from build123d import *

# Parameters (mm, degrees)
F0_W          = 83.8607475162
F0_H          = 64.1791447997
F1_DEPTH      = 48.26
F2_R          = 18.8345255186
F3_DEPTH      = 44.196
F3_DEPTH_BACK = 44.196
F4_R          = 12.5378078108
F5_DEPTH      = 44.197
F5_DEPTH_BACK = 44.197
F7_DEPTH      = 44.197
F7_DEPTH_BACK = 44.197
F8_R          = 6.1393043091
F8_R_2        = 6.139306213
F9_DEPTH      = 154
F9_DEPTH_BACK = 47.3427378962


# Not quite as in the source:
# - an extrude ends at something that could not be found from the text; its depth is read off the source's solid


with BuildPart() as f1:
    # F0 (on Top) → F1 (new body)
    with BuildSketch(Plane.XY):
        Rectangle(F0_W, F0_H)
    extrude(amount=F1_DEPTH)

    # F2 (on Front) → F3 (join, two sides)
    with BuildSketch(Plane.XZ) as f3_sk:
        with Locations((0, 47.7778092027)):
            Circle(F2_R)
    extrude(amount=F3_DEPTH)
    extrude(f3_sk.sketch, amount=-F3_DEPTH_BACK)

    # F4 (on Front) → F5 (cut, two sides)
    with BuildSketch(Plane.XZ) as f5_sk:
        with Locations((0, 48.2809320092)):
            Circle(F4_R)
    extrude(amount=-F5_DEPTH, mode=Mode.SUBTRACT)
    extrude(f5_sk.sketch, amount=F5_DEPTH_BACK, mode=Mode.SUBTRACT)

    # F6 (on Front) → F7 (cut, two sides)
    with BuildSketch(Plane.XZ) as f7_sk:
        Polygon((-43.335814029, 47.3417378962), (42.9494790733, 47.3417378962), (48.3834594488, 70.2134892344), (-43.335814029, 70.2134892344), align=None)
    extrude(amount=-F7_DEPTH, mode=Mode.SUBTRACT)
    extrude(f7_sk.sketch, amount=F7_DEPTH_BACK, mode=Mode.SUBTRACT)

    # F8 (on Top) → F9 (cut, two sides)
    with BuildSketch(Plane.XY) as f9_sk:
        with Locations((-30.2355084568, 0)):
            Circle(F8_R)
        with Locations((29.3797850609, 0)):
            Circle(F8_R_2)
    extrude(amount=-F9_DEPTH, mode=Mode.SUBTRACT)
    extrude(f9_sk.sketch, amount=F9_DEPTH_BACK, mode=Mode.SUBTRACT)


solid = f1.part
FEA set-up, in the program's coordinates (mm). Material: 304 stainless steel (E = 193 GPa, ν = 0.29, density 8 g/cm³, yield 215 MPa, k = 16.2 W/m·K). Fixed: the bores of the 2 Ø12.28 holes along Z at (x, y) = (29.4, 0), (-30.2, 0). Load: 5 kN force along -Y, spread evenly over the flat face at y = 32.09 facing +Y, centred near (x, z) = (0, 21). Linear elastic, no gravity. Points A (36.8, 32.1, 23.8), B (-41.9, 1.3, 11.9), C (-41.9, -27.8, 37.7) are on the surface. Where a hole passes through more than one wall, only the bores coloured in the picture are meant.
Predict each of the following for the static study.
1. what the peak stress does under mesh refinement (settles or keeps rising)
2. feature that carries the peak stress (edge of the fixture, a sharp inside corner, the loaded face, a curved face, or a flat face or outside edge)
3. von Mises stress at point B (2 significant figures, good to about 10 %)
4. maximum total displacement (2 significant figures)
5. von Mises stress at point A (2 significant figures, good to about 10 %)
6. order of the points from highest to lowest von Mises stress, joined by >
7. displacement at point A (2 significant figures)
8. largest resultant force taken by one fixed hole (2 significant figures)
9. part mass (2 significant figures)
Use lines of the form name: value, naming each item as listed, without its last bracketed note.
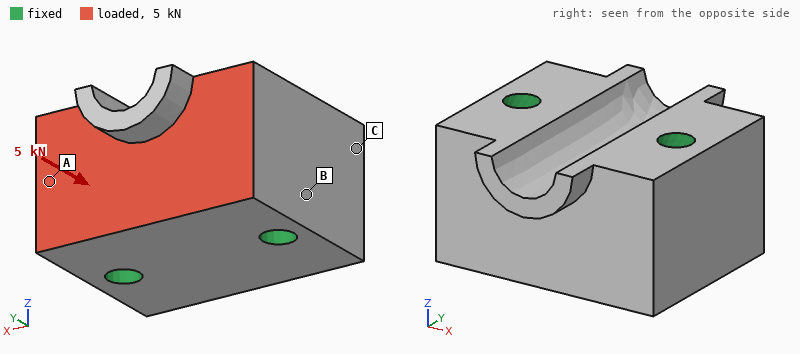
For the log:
what the peak stress does under mesh refinement: keeps rising
feature that carries the peak stress: edge of the fixture
von Mises stress at point B: 0.87 MPa
maximum total displacement: 0.39 µm
von Mises stress at point A: 1.5 MPa
order of the points from highest to lowest von Mises stress, joined by >: A > B > C
displacement at point A: 0.23 µm
largest resultant force taken by one fixed hole: 2.5 kN
part mass: 1.9 kg
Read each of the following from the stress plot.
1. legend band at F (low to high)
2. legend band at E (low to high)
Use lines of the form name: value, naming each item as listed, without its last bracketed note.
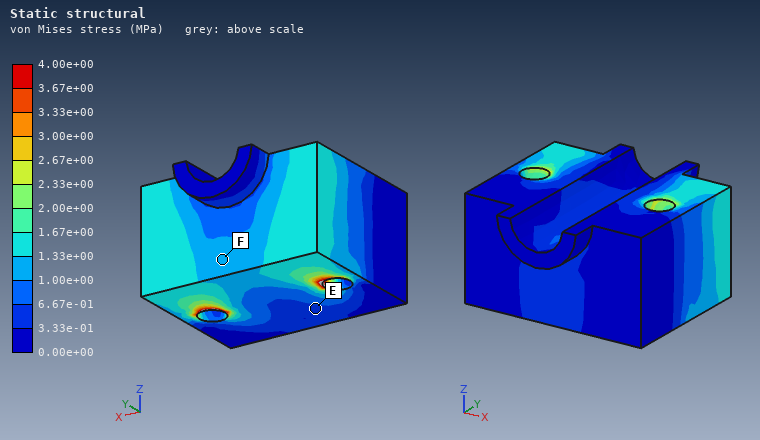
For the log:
legend band at F: 1.00e+00 to 1.33e+00 MPa
legend band at E: 3.33e-01 to 6.67e-01 MPa
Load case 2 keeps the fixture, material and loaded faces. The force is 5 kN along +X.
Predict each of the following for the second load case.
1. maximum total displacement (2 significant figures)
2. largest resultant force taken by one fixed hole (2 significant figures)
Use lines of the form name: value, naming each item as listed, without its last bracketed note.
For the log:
maximum total displacement: 1.2 µm
largest resultant force taken by one fixed hole: 3.3 kN
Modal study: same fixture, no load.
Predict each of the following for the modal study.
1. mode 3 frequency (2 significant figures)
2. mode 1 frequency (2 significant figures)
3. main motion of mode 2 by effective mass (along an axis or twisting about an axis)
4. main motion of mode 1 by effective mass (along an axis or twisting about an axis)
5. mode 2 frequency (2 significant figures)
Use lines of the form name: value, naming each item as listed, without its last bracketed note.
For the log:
mode 3 frequency: 19 kHz
mode 1 frequency: 15 kHz
main motion of mode 2 by effective mass: along Z
main motion of mode 1 by effective mass: twisting about X
mode 2 frequency: 16 kHz
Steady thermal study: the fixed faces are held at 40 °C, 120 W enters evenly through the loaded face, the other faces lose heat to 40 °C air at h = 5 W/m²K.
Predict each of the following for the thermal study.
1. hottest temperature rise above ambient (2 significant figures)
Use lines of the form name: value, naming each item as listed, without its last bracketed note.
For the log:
hottest temperature rise above ambient: 69 K
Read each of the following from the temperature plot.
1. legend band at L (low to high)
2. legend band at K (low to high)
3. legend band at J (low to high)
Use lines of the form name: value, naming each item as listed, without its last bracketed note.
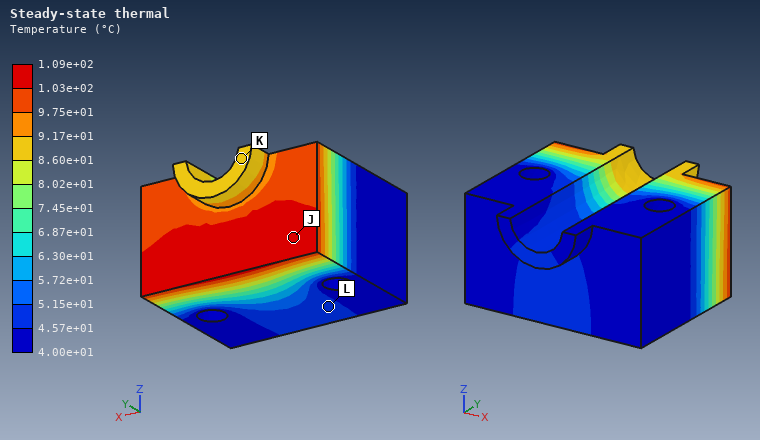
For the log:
legend band at L: 4.57e+01 to 5.15e+01 °C
legend band at K: 8.60e+01 to 9.17e+01 °C
legend band at J: 1.03e+02 to 1.09e+02 °C
